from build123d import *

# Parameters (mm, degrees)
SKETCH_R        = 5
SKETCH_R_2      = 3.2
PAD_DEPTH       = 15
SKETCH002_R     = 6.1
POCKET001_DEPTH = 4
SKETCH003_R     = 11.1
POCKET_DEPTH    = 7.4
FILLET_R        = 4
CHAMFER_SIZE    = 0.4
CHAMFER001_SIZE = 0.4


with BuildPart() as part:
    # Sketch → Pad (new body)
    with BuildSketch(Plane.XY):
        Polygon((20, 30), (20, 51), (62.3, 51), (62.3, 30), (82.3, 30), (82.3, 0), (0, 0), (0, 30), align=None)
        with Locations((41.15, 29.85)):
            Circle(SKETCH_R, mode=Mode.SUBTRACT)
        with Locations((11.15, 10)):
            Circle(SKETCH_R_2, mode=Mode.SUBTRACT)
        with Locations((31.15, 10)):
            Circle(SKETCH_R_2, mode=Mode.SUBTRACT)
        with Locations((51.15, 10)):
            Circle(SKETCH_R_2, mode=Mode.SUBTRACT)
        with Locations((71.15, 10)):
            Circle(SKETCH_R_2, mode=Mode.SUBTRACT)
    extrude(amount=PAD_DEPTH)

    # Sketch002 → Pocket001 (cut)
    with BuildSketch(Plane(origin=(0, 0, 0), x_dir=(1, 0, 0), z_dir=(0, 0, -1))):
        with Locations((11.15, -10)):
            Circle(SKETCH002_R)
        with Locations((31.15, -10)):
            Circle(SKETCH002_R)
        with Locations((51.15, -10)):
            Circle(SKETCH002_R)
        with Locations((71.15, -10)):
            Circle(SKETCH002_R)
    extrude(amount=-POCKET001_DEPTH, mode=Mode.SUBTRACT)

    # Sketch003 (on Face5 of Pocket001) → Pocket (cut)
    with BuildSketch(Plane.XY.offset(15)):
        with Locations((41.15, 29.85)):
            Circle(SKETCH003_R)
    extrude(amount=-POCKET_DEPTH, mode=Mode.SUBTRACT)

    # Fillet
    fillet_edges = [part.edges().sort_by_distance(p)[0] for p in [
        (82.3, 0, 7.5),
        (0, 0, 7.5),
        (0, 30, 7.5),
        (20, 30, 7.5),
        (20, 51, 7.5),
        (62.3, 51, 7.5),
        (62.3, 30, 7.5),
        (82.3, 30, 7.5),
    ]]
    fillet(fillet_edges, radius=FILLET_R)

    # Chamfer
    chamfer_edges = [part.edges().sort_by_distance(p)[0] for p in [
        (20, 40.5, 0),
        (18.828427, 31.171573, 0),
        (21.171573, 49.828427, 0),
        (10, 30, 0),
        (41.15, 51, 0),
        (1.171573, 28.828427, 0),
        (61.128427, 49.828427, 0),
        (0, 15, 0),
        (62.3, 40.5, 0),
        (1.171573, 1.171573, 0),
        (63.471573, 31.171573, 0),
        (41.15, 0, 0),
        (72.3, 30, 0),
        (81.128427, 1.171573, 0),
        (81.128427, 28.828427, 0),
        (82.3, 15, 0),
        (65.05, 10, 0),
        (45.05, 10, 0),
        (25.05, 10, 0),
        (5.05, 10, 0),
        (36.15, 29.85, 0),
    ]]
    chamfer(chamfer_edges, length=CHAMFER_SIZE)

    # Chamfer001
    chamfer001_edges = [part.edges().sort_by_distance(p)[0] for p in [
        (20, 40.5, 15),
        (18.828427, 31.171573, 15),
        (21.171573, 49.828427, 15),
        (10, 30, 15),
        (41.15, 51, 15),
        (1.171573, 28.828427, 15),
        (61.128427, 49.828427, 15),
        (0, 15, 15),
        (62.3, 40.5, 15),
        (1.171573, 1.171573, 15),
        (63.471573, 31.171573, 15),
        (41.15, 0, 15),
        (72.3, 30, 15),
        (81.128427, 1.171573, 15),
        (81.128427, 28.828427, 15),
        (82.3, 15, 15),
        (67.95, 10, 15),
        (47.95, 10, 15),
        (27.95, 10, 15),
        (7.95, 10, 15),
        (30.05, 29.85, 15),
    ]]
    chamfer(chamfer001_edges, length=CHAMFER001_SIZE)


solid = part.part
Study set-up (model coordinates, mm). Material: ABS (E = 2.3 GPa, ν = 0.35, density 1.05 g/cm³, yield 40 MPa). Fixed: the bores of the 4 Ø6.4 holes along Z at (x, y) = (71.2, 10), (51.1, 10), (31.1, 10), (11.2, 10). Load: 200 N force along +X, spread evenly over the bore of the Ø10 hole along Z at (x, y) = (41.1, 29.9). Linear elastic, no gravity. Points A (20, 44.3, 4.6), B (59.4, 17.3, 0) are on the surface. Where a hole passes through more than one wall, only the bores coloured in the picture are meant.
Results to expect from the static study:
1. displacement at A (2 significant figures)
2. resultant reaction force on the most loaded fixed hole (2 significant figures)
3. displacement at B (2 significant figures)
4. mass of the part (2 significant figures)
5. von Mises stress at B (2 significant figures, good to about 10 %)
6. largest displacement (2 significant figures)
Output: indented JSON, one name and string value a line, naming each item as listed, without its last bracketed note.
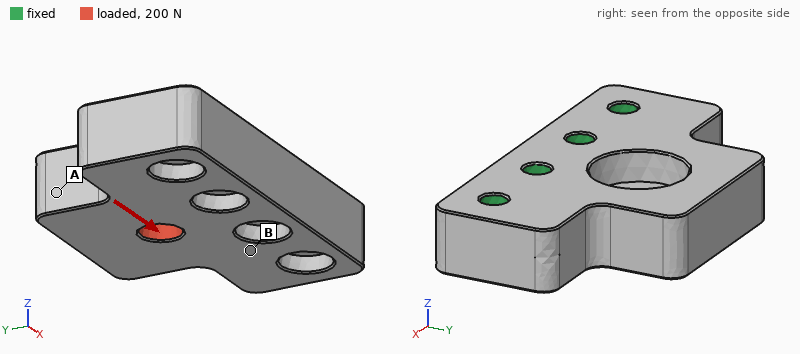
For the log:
{
  "displacement at A": "9.1 µm",
  "resultant reaction force on the most loaded fixed hole": "75 N",
  "displacement at B": "2.4 µm",
  "mass of the part": "46 g",
  "von Mises stress at B": "0.32 MPa",
  "largest displacement": "12 µm"
}
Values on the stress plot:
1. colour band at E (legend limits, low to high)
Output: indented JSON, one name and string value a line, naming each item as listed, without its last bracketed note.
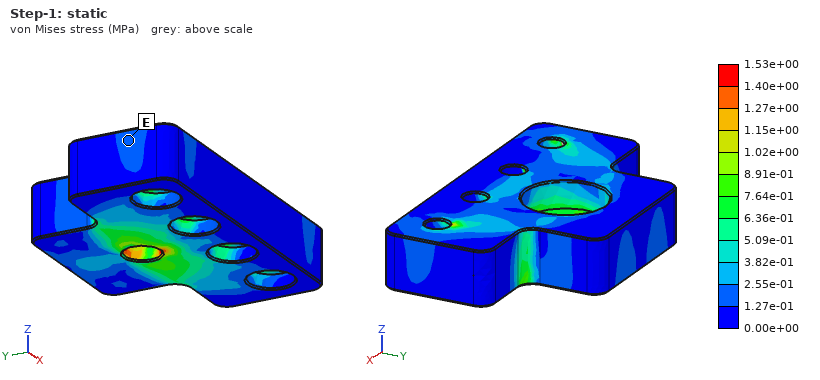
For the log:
{
  "colour band at E": "1.27e-01 to 2.55e-01 MPa"
}
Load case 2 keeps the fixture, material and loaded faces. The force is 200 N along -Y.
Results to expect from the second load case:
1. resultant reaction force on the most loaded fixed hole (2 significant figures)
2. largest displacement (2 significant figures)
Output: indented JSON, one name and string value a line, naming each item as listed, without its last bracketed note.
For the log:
{
  "resultant reaction force on the most loaded fixed hole": "76 N",
  "largest displacement": "21 µm"
}
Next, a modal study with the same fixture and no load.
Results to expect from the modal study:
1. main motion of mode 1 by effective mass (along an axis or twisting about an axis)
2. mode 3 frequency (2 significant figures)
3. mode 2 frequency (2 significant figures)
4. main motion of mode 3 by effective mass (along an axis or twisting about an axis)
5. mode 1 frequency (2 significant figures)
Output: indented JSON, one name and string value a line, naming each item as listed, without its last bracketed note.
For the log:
{
  "main motion of mode 1 by effective mass": "along Z",
  "mode 3 frequency": "5000 Hz",
  "mode 2 frequency": "3700 Hz",
  "main motion of mode 3 by effective mass": "along X",
  "mode 1 frequency": "1900 Hz"
}
